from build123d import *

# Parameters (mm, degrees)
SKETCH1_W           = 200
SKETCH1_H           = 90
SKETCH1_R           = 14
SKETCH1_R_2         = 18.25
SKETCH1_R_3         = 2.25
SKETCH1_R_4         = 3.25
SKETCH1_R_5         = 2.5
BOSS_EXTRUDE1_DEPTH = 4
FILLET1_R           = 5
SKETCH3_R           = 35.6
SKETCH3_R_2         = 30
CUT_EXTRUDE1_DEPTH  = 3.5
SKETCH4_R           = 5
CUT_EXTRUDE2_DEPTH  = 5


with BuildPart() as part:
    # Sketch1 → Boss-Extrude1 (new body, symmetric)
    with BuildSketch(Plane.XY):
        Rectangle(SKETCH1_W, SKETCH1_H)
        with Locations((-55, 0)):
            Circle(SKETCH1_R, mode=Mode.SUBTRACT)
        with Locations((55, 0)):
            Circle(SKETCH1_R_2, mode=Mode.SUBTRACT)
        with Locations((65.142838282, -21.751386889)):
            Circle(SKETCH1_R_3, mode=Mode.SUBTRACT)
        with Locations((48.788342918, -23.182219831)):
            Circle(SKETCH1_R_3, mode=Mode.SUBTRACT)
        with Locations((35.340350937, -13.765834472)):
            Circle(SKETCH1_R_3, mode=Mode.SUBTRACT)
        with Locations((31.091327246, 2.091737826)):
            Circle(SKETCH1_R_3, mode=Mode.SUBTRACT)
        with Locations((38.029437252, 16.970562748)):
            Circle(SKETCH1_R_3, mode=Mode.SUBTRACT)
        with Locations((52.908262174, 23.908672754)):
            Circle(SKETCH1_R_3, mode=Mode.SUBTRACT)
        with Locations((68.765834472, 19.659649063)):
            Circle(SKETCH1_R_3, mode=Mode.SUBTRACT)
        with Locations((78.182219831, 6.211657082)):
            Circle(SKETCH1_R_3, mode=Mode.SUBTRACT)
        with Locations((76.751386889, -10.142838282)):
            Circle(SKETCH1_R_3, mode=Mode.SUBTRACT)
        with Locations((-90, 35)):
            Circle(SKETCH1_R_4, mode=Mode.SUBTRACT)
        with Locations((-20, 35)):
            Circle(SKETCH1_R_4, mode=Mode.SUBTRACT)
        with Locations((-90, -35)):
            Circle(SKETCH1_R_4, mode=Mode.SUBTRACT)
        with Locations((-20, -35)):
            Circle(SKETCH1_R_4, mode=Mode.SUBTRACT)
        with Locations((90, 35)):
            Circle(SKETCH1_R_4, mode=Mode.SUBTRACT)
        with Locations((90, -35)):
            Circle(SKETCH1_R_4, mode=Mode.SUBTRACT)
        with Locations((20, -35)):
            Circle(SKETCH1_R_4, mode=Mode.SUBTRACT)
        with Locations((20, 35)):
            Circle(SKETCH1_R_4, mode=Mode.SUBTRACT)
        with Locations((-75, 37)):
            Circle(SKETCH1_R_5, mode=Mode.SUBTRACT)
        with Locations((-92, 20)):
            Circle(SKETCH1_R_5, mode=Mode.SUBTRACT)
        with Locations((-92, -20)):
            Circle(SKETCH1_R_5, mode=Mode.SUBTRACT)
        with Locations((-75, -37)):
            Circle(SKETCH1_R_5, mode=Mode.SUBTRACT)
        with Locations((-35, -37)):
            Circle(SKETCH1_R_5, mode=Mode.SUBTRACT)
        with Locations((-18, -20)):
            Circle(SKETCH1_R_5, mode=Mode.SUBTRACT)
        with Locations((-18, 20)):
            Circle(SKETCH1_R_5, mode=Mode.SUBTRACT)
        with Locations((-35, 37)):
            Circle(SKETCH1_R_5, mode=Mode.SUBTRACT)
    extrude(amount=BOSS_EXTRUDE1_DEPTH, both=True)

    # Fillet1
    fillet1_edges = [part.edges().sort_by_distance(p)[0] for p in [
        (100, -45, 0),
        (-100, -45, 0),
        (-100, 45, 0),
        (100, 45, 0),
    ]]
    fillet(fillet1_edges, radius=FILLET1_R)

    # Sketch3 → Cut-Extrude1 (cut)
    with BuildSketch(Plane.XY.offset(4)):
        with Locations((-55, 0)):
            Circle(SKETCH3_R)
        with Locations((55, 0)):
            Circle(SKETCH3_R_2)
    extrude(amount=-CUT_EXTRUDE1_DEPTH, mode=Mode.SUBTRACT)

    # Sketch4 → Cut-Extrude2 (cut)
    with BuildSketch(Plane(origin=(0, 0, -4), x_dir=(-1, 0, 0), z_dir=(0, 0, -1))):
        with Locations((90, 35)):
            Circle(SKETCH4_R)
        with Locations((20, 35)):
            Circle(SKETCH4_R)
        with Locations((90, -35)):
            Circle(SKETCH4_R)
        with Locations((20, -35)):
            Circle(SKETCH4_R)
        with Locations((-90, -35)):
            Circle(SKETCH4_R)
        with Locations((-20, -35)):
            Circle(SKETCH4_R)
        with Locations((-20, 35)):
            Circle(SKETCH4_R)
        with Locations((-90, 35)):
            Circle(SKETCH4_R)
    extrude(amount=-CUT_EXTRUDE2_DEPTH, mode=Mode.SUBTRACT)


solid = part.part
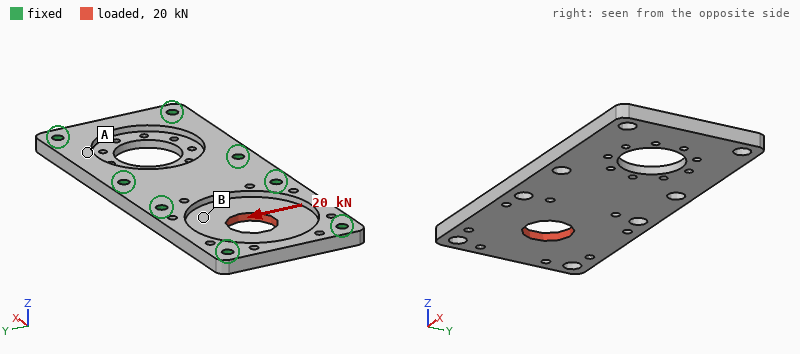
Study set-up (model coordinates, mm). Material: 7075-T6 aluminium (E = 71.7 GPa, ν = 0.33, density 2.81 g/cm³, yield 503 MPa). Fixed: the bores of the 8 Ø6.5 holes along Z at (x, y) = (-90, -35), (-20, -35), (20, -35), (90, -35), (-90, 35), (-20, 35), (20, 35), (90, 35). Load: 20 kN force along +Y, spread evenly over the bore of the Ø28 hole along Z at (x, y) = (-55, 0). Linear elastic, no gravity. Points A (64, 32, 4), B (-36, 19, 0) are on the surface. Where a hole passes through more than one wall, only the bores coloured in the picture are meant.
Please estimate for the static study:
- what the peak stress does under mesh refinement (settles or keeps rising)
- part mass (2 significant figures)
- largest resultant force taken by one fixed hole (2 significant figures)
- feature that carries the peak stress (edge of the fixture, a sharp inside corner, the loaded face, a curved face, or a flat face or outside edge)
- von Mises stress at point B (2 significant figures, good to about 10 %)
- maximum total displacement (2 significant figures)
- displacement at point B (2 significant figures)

keeps rising
300 g
5.1 kN
edge of the fixture
58 MPa
53 µm
34 µm
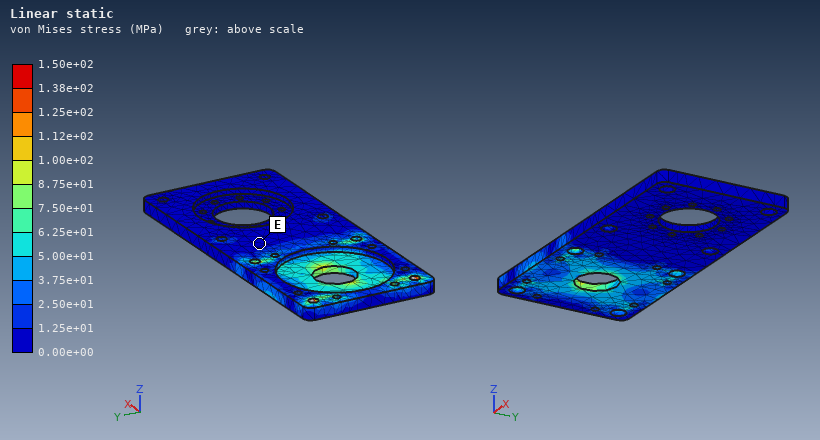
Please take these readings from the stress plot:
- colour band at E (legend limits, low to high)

0.00e+00 to 1.25e+01 MPa
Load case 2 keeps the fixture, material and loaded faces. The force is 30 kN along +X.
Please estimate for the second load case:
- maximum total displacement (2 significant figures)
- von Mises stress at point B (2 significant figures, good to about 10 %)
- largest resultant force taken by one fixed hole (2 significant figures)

81 µm
87 MPa
6.0 kN
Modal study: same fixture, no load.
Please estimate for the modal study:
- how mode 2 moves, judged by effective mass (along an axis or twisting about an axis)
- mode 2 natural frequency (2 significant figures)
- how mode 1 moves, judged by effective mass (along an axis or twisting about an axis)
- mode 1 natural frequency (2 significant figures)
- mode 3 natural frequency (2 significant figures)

along Z
5600 Hz
along Z
5100 Hz
6300 Hz
